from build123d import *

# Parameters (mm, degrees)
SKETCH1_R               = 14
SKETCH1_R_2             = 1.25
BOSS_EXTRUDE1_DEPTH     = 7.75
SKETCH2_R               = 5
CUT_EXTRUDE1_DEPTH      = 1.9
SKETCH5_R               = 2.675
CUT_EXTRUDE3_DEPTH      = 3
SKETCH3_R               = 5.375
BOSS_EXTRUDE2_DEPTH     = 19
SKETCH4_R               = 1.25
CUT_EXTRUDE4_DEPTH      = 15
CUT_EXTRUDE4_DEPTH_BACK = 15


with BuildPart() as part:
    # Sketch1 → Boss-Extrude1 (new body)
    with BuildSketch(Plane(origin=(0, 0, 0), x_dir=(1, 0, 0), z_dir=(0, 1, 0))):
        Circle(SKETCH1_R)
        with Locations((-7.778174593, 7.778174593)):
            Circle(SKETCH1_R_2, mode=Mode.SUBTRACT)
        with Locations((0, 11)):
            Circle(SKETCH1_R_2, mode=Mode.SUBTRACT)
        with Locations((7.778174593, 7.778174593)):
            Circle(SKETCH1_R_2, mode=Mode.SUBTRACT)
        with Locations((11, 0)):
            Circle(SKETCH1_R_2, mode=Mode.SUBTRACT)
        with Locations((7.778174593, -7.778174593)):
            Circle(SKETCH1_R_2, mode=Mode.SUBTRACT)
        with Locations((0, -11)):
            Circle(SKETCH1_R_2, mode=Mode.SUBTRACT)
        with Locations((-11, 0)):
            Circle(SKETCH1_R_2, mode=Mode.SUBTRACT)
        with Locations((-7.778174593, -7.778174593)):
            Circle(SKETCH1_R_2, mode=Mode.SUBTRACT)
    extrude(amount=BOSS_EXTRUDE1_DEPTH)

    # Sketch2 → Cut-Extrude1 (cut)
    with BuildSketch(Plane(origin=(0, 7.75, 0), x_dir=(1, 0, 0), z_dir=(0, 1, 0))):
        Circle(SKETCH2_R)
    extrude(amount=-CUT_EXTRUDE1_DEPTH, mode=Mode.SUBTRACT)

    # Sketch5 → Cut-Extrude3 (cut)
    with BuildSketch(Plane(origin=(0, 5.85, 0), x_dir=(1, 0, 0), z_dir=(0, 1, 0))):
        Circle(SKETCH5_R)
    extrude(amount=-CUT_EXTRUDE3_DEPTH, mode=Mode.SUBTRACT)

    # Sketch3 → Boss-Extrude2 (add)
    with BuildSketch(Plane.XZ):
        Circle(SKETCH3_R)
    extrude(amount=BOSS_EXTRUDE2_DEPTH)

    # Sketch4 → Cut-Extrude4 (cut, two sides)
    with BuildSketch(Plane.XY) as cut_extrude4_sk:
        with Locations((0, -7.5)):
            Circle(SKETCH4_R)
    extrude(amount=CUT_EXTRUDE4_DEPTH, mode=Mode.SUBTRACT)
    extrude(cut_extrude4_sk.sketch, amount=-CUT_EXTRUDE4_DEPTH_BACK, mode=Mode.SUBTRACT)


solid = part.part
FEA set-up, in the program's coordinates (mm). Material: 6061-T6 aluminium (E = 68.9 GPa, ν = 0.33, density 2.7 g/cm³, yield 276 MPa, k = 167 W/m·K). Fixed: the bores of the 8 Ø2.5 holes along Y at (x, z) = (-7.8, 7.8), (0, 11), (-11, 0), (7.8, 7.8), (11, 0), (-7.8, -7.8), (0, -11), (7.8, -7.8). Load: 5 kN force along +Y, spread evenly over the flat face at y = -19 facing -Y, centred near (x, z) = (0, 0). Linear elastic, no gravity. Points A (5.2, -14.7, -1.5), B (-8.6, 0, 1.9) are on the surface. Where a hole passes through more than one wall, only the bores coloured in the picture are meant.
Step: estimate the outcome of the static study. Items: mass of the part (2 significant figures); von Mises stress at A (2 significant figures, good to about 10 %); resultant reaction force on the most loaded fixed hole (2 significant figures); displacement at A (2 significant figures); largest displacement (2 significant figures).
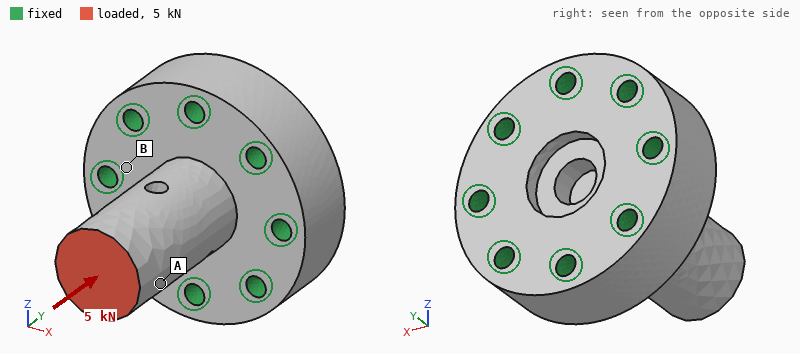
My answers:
16 g
59 MPa
740 N
19 µm
23 µm
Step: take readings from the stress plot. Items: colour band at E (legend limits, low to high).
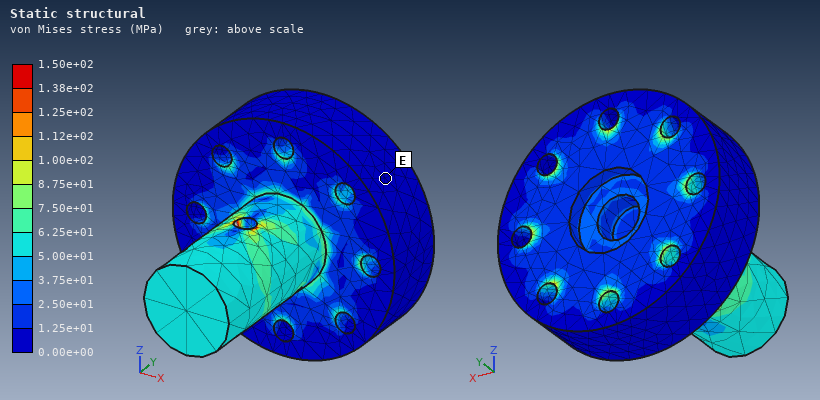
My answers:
0.00e+00 to 1.25e+01 MPa
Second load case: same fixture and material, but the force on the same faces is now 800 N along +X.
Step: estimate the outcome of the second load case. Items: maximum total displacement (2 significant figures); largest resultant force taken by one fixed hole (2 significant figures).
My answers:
74 µm
550 N
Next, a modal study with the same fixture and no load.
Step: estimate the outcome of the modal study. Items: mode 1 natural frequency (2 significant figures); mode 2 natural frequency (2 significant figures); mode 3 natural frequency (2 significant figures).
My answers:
14 kHz
14 kHz
37 kHz
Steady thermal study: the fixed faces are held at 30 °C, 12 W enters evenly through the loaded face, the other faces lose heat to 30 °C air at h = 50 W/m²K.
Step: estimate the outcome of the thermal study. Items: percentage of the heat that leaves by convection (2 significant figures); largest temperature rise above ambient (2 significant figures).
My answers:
3.3 %
18 K
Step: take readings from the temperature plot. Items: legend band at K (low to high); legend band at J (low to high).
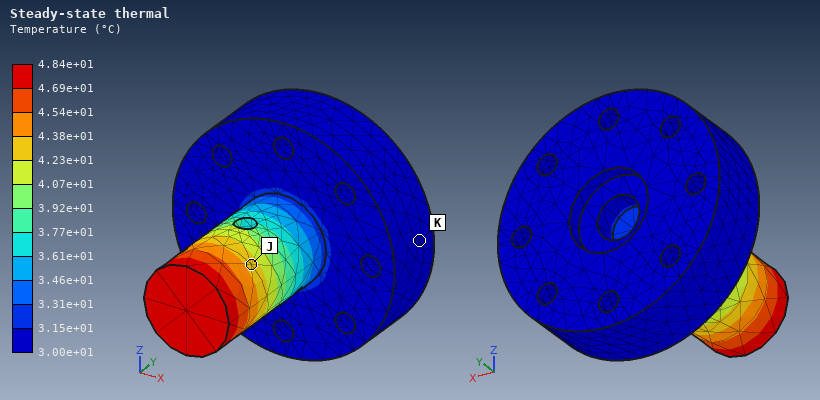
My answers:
3.00e+01 to 3.15e+01 °C
4.23e+01 to 4.38e+01 °C
